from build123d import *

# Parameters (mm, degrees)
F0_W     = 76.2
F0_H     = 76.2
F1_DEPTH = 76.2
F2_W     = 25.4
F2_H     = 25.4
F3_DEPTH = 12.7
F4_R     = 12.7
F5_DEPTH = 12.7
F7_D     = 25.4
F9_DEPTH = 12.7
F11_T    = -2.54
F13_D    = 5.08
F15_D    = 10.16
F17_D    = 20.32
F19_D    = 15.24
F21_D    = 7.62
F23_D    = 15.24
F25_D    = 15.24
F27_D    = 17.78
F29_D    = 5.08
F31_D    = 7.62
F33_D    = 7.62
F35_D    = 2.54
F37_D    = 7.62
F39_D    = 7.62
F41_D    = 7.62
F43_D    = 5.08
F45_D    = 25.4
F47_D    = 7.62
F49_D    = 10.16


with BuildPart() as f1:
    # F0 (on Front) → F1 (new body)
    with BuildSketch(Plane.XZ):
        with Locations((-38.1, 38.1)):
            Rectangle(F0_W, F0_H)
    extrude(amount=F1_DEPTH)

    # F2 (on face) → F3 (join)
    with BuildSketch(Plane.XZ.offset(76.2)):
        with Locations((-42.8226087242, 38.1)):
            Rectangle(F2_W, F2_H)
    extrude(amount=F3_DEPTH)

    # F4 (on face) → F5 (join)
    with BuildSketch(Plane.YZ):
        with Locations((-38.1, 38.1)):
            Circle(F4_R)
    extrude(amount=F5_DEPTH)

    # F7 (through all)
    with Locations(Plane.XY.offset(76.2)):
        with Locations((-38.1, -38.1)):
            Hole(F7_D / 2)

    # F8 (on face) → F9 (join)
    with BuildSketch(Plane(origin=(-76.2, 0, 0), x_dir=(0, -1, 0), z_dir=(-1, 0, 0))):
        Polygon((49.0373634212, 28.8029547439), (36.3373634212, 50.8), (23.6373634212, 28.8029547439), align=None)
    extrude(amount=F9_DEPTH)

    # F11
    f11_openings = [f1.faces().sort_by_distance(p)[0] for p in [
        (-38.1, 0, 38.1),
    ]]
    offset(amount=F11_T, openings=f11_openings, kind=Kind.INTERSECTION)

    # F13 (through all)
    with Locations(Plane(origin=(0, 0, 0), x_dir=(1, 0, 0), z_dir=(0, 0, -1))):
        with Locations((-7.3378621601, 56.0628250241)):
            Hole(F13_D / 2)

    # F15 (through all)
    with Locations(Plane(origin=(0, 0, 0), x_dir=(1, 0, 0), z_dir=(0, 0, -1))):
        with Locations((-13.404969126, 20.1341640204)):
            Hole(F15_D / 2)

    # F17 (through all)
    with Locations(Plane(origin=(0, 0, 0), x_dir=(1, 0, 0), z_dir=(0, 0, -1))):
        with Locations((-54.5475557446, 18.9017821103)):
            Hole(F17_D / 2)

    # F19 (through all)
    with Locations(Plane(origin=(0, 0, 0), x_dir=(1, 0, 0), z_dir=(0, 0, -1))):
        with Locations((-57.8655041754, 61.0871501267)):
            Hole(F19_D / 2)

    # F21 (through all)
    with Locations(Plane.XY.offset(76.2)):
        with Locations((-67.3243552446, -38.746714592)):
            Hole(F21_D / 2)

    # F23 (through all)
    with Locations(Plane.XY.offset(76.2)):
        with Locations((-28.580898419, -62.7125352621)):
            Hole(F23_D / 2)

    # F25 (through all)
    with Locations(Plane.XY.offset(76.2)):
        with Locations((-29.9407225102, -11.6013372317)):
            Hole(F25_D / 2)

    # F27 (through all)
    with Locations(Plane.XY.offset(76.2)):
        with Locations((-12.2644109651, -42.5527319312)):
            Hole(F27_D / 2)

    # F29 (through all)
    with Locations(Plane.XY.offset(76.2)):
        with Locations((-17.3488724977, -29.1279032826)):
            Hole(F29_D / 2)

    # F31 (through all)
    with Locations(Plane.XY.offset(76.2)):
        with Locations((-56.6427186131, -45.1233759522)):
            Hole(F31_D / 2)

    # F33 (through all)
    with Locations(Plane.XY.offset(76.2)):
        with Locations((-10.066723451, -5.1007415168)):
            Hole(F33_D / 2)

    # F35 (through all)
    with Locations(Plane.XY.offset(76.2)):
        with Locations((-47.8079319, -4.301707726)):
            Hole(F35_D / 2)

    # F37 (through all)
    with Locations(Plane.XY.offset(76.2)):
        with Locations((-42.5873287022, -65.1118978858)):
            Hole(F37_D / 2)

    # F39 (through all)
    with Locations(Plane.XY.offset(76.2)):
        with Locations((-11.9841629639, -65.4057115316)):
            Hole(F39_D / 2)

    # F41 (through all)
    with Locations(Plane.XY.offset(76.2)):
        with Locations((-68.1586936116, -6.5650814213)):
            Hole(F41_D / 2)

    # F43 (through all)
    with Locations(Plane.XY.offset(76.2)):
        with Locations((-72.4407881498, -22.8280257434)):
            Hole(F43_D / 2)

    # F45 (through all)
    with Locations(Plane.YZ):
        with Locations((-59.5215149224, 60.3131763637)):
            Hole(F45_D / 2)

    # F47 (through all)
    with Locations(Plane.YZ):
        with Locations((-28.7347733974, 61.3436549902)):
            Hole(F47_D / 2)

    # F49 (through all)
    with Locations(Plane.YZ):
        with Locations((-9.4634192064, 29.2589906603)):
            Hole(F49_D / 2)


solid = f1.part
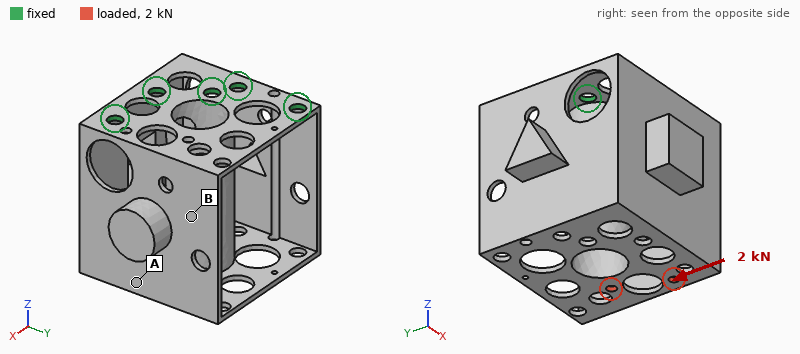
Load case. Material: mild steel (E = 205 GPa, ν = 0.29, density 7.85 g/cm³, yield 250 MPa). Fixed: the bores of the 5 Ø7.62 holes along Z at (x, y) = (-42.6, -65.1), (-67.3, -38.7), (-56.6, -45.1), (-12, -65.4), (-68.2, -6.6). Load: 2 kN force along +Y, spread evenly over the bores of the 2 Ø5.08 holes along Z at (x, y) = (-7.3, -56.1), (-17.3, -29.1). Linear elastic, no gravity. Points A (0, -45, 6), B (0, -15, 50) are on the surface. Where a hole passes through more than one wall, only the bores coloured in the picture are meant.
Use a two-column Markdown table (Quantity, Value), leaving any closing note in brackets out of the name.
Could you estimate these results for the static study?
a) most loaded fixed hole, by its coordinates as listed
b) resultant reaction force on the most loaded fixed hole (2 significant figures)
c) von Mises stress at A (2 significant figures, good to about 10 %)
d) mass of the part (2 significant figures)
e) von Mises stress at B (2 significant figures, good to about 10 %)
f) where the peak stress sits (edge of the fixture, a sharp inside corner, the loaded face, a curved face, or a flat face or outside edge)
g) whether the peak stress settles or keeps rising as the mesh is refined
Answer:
| Quantity | Value |
|---|---|
| most loaded fixed hole, by its coordinates as listed | (-68.2, -6.6) |
| resultant reaction force on the most loaded fixed hole | 2.7 kN |
| von Mises stress at A | 40 MPa |
| mass of the part | 610 g |
| von Mises stress at B | 21 MPa |
| where the peak stress sits | edge of the fixture |
| whether the peak stress settles or keeps rising as the mesh is refined | keeps rising |
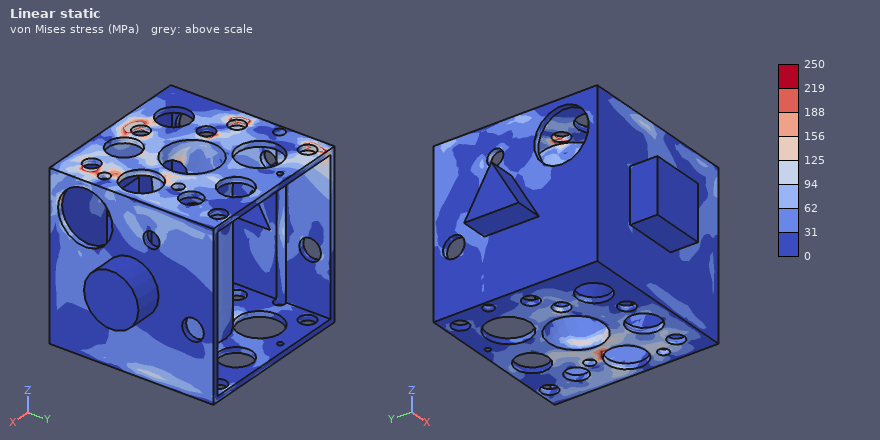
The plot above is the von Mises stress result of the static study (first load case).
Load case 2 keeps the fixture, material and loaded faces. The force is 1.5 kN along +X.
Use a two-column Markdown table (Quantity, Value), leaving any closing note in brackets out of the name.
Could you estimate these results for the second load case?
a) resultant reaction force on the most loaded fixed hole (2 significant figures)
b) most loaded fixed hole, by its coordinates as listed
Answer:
| Quantity | Value |
|---|---|
| resultant reaction force on the most loaded fixed hole | 2.3 kN |
| most loaded fixed hole, by its coordinates as listed | (-12, -65.4) |
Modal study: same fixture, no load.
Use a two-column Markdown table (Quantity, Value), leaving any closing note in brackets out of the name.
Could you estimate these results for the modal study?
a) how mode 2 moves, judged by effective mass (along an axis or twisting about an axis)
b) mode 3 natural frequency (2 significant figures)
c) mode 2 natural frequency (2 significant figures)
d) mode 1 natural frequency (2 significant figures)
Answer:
| Quantity | Value |
|---|---|
| how mode 2 moves, judged by effective mass | along X |
| mode 3 natural frequency | 1900 Hz |
| mode 2 natural frequency | 1100 Hz |
| mode 1 natural frequency | 900 Hz |
